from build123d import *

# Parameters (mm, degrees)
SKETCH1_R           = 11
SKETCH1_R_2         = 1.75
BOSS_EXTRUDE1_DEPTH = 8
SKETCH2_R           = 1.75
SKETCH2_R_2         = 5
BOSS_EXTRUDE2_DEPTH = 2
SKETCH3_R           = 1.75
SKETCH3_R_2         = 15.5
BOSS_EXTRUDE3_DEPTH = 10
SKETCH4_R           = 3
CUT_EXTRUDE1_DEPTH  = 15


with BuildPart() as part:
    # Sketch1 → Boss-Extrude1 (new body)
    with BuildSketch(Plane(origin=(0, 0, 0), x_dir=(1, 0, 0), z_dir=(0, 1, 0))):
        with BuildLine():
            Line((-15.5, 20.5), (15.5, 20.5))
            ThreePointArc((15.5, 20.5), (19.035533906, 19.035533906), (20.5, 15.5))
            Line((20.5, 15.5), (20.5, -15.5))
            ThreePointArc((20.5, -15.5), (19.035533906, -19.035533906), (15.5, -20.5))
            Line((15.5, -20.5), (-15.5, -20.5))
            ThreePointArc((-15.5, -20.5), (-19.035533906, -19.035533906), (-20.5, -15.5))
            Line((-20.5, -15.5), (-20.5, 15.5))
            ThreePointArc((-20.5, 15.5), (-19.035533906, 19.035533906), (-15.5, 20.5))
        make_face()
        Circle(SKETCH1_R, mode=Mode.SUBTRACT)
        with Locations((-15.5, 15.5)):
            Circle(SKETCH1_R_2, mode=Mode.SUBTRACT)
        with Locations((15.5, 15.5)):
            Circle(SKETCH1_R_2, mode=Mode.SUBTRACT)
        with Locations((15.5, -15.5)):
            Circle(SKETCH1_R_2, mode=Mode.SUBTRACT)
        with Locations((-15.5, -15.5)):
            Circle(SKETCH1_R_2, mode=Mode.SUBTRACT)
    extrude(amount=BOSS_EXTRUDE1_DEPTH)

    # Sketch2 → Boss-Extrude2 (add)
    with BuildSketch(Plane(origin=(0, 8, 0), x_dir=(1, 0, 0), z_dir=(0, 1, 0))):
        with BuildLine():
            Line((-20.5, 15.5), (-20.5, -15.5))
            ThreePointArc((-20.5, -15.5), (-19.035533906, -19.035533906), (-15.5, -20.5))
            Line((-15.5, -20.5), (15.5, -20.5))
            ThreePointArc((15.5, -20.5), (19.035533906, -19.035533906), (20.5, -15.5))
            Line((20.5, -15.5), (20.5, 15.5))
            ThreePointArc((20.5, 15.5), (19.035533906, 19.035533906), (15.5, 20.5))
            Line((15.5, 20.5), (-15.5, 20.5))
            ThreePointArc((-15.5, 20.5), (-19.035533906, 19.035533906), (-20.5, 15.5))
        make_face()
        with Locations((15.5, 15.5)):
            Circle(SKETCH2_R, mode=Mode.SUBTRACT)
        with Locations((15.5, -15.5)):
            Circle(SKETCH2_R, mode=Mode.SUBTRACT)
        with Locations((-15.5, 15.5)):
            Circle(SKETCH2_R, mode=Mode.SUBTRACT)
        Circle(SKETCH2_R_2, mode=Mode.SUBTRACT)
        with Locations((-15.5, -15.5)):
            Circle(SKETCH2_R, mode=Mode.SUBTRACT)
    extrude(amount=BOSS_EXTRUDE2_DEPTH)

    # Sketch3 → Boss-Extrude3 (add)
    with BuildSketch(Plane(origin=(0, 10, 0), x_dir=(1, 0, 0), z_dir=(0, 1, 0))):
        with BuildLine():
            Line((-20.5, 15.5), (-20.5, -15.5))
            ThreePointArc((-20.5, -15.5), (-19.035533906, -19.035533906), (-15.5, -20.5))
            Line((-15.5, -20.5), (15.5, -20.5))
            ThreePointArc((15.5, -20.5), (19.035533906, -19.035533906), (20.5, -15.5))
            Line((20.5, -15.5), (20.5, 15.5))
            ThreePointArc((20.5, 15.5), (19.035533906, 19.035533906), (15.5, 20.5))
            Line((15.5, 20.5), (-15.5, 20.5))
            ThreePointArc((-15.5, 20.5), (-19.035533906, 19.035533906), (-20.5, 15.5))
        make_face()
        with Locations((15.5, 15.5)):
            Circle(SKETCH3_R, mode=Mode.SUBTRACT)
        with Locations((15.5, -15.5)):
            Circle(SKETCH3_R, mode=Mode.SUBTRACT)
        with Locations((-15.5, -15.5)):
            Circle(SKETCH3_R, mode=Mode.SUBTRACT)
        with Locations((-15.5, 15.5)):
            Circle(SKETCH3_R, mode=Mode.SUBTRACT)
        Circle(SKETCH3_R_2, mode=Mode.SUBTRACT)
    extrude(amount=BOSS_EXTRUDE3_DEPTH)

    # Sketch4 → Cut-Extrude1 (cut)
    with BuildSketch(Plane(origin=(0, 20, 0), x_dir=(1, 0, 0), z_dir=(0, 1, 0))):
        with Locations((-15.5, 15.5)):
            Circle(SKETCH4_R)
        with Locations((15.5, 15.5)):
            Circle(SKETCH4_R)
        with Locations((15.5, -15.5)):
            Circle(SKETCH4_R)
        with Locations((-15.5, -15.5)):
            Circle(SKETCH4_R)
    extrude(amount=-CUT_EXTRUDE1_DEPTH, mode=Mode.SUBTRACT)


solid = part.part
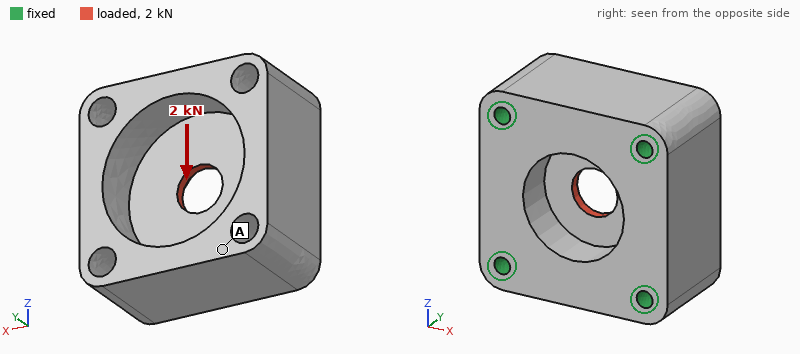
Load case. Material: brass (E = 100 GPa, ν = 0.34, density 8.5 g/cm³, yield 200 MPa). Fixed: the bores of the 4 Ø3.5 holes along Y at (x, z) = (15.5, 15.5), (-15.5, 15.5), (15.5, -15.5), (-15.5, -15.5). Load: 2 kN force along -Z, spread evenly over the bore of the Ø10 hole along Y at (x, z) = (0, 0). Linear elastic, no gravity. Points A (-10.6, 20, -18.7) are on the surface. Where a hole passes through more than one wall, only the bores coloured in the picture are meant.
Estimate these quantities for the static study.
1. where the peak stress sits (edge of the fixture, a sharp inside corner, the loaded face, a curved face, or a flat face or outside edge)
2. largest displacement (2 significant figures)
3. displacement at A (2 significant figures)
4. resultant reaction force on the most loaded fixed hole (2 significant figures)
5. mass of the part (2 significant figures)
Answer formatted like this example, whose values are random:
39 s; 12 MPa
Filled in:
the loaded face; 4.4 µm; 1.4 µm; 550 N; 170 g
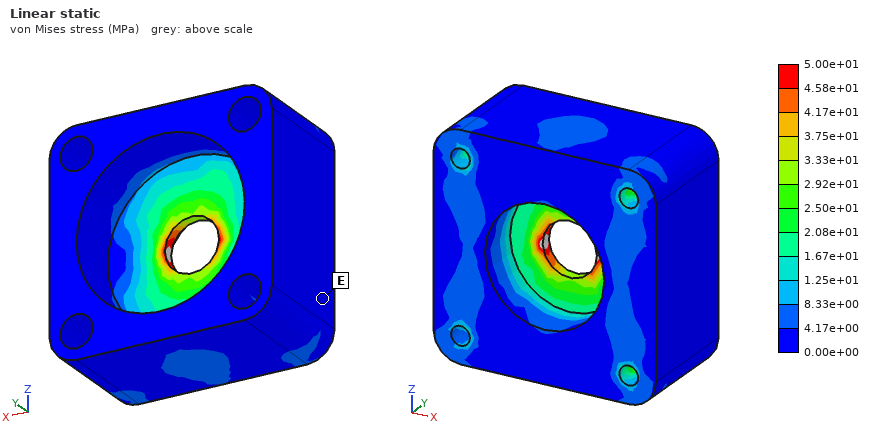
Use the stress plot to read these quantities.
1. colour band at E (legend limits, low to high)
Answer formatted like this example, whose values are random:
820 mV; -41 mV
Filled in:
0.00e+00 to 4.17e+00 MPa
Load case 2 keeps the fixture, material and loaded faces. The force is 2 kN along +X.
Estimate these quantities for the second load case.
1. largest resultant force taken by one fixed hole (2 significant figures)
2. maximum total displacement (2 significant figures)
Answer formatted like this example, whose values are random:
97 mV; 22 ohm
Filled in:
550 N; 4.4 µm
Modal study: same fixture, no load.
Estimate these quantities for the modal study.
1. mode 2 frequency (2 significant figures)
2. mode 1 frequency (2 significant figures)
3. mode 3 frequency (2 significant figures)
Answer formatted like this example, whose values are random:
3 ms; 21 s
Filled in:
15 kHz; 14 kHz; 15 kHz
